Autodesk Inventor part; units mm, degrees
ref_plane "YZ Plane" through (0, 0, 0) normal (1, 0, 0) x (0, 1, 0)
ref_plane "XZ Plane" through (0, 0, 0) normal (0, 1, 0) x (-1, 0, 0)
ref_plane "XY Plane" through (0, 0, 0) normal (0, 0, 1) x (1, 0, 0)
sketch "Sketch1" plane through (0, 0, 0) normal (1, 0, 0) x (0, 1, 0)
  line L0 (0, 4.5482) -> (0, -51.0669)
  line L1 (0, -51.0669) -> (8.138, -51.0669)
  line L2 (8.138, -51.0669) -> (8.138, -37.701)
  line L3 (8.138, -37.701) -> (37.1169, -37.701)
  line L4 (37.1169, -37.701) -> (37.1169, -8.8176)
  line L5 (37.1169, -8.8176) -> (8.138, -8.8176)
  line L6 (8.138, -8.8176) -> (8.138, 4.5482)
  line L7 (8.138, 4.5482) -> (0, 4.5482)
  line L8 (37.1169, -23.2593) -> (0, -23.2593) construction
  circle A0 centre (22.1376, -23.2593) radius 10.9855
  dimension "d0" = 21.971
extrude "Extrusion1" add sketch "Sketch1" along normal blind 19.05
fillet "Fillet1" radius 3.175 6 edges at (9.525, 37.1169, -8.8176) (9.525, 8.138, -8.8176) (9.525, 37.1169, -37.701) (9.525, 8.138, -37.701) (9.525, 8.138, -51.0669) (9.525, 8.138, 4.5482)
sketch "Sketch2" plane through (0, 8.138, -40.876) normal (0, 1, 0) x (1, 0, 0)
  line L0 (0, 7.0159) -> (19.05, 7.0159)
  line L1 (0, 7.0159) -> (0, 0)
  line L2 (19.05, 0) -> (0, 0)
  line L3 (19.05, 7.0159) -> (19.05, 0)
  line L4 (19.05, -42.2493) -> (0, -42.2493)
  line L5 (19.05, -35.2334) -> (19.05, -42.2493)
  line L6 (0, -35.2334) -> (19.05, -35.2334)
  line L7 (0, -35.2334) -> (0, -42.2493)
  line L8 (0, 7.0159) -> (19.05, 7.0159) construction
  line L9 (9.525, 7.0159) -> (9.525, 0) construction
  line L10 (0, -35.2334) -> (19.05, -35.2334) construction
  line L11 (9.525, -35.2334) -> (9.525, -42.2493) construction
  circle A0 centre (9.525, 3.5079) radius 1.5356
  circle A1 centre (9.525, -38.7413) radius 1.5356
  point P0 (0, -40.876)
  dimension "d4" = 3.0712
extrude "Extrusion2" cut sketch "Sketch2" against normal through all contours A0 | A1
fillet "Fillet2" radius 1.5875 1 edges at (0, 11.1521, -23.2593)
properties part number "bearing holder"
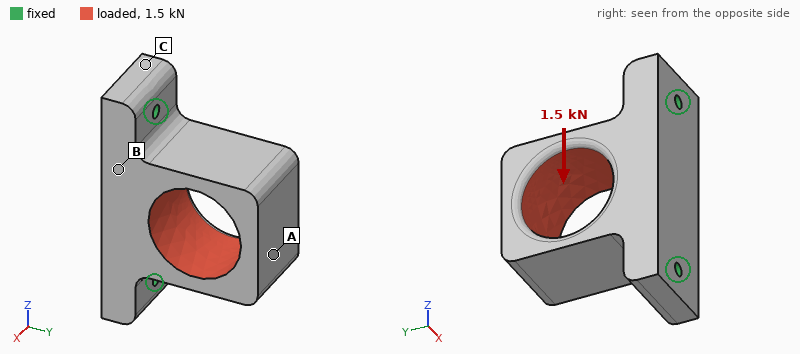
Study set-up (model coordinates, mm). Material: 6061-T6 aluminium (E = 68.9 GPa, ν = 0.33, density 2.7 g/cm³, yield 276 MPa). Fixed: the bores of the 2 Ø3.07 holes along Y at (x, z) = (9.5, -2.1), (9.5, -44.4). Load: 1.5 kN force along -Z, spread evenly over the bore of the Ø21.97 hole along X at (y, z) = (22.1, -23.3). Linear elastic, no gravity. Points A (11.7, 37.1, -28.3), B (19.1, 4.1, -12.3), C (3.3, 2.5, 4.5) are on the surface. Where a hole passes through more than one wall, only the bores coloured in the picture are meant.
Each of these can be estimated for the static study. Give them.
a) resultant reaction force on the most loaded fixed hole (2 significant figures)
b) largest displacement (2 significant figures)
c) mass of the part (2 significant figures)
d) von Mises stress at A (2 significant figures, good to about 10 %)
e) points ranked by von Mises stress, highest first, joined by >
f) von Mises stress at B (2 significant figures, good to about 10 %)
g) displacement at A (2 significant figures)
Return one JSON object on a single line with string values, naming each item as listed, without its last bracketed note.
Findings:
{"resultant reaction force on the most loaded fixed hole": "1.0 kN", "largest displacement": "33 µm", "mass of the part": "46 g", "von Mises stress at A": "12 MPa", "points ranked by von Mises stress, highest first, joined by >": "A > B > C", "von Mises stress at B": "6.5 MPa", "displacement at A": "31 µm"}
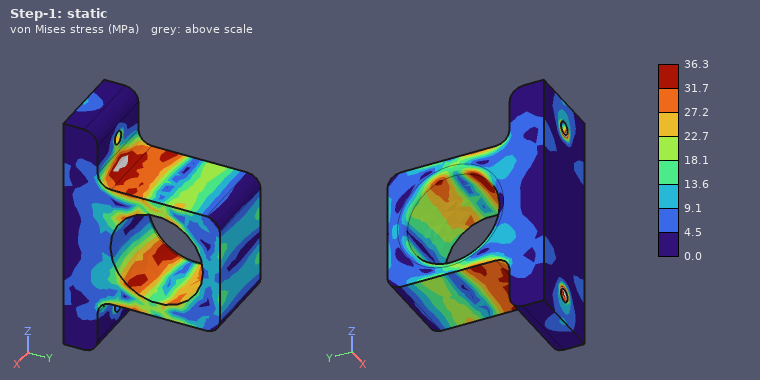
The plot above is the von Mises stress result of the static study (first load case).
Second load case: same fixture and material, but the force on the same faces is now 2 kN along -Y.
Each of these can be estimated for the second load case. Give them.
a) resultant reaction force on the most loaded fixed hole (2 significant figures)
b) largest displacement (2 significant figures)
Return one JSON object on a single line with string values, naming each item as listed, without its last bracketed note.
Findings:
{"resultant reaction force on the most loaded fixed hole": "1.1 kN", "largest displacement": "14 µm"}
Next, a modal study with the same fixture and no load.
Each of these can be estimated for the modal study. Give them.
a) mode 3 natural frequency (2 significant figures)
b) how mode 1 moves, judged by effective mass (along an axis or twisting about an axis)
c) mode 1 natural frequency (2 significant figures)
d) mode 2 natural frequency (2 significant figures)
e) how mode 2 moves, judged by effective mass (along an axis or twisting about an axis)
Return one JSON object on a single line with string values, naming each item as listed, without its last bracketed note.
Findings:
{"mode 3 natural frequency": "12 kHz", "how mode 1 moves, judged by effective mass": "along X", "mode 1 natural frequency": "4800 Hz", "mode 2 natural frequency": "7500 Hz", "how mode 2 moves, judged by effective mass": "along Z"}
